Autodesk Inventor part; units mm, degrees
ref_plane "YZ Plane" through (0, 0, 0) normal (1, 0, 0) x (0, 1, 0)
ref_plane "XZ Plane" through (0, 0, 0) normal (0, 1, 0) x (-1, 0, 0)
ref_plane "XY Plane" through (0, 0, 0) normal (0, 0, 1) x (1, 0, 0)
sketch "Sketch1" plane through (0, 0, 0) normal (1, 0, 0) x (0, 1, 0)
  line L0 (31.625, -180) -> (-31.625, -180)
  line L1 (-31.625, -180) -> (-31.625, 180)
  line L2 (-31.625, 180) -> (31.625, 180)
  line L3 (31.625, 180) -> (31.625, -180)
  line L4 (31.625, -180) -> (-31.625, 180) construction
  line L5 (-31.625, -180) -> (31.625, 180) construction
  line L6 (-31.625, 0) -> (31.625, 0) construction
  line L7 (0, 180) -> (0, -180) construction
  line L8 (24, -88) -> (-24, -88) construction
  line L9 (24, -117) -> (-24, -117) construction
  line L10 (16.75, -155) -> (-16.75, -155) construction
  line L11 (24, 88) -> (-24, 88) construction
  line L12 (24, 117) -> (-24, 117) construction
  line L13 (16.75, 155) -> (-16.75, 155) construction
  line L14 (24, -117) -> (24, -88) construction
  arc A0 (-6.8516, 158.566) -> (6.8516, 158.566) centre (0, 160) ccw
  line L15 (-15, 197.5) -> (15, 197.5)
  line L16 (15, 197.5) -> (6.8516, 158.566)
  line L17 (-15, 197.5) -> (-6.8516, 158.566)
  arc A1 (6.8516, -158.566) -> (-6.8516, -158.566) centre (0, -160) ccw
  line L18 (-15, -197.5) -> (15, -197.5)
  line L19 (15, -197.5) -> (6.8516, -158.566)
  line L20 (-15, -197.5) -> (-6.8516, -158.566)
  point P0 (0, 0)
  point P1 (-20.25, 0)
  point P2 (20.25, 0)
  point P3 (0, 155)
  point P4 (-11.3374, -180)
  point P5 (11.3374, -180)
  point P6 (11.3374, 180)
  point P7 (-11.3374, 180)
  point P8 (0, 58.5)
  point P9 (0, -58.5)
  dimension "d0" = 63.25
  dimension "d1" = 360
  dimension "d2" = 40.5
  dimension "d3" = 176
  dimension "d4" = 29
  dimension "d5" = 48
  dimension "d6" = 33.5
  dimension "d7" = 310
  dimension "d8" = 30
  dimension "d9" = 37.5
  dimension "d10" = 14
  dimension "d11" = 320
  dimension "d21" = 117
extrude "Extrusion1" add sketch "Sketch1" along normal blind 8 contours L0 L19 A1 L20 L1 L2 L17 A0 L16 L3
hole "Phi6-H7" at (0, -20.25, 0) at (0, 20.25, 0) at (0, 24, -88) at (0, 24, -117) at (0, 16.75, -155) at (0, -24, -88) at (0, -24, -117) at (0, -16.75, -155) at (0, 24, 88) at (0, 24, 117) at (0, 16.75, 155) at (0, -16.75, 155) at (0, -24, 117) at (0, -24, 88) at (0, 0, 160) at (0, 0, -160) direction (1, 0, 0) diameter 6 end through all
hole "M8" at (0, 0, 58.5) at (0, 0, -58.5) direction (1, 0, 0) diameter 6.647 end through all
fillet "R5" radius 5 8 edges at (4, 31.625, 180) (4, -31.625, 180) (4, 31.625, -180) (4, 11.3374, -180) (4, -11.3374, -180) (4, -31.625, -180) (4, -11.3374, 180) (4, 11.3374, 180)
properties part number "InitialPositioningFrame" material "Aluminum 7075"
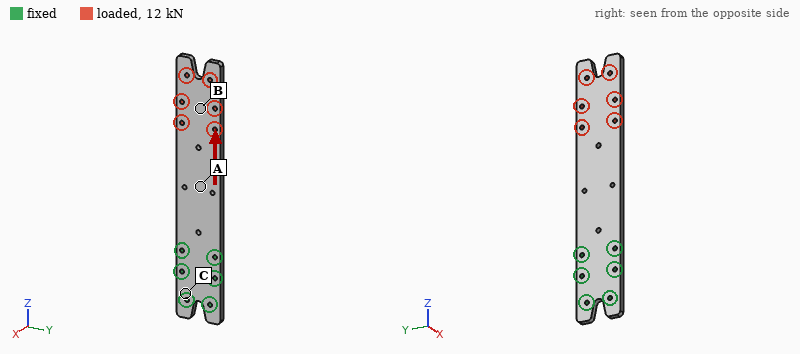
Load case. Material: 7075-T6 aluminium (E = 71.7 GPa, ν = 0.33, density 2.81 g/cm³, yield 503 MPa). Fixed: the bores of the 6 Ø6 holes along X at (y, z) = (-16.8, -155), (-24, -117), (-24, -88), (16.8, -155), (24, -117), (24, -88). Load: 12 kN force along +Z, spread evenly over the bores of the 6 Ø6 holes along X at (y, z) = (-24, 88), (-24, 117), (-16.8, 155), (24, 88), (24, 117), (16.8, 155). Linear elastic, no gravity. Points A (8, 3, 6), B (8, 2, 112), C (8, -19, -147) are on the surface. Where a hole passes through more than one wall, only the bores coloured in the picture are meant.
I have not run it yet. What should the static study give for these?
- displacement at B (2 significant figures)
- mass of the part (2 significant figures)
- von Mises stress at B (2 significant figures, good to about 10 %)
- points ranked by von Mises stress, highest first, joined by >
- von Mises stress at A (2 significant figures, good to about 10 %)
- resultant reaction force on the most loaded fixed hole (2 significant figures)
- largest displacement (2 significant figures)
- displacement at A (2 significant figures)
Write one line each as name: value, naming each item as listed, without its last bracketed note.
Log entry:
displacement at B: 67 µm
mass of the part: 480 g
von Mises stress at B: 14 MPa
points ranked by von Mises stress, highest first, joined by >: A > B > C
von Mises stress at A: 24 MPa
resultant reaction force on the most loaded fixed hole: 4.8 kN
largest displacement: 76 µm
displacement at A: 34 µm
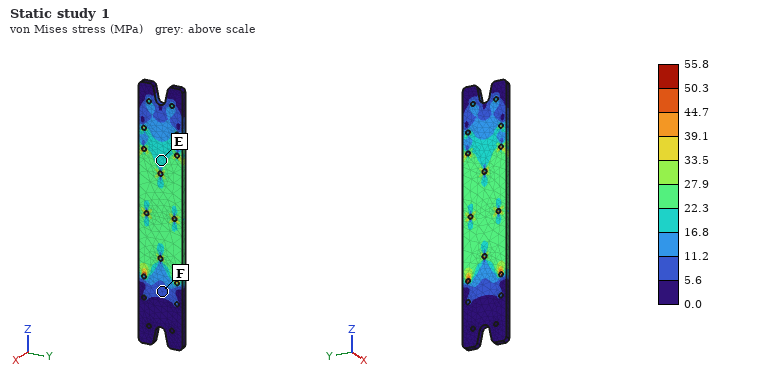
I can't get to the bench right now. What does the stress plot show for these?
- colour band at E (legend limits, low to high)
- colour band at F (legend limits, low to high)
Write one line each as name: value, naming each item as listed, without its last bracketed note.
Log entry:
colour band at E: 16.8 to 22.3 MPa
colour band at F: 5.6 to 11.2 MPa
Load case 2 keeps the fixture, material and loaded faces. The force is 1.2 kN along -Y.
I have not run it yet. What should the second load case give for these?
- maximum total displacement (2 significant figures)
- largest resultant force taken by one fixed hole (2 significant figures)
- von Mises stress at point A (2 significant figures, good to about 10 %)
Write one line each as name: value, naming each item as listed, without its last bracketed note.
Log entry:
maximum total displacement: 0.47 mm
largest resultant force taken by one fixed hole: 4.7 kN
von Mises stress at point A: 7.7 MPa
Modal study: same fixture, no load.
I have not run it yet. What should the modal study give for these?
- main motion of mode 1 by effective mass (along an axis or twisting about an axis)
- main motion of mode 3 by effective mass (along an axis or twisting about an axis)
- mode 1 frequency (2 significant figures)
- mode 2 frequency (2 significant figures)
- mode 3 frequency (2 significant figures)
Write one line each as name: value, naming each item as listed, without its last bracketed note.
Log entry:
main motion of mode 1 by effective mass: along X
main motion of mode 3 by effective mass: along Y
mode 1 frequency: 95 Hz
mode 2 frequency: 580 Hz
mode 3 frequency: 720 Hz
